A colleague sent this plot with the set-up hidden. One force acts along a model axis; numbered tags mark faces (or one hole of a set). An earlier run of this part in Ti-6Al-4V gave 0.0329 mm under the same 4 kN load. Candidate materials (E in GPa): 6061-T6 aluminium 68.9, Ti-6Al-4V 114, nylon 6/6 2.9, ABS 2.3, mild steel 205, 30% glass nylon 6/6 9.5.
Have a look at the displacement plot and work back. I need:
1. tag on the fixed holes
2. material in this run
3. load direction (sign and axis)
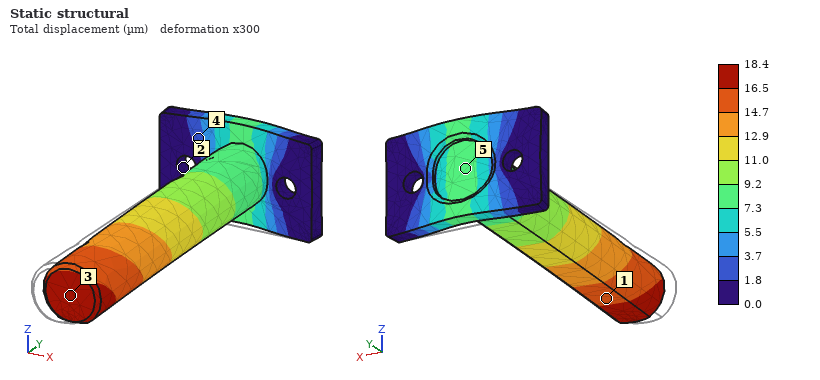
2
mild steel
+Y
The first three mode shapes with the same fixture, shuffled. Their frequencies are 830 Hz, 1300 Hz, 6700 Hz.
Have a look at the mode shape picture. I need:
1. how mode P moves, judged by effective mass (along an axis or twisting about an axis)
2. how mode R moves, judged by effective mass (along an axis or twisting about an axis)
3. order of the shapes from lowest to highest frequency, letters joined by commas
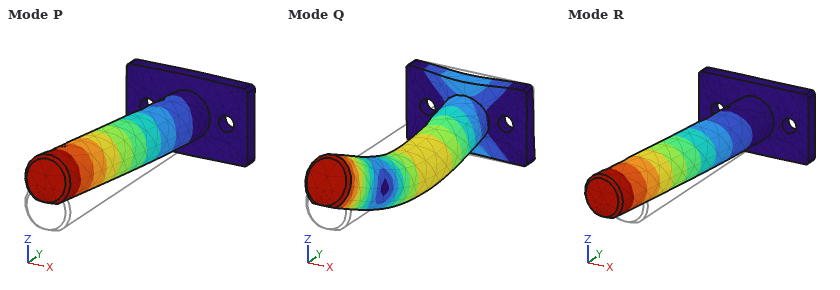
along Z
along X
P, R, Q
